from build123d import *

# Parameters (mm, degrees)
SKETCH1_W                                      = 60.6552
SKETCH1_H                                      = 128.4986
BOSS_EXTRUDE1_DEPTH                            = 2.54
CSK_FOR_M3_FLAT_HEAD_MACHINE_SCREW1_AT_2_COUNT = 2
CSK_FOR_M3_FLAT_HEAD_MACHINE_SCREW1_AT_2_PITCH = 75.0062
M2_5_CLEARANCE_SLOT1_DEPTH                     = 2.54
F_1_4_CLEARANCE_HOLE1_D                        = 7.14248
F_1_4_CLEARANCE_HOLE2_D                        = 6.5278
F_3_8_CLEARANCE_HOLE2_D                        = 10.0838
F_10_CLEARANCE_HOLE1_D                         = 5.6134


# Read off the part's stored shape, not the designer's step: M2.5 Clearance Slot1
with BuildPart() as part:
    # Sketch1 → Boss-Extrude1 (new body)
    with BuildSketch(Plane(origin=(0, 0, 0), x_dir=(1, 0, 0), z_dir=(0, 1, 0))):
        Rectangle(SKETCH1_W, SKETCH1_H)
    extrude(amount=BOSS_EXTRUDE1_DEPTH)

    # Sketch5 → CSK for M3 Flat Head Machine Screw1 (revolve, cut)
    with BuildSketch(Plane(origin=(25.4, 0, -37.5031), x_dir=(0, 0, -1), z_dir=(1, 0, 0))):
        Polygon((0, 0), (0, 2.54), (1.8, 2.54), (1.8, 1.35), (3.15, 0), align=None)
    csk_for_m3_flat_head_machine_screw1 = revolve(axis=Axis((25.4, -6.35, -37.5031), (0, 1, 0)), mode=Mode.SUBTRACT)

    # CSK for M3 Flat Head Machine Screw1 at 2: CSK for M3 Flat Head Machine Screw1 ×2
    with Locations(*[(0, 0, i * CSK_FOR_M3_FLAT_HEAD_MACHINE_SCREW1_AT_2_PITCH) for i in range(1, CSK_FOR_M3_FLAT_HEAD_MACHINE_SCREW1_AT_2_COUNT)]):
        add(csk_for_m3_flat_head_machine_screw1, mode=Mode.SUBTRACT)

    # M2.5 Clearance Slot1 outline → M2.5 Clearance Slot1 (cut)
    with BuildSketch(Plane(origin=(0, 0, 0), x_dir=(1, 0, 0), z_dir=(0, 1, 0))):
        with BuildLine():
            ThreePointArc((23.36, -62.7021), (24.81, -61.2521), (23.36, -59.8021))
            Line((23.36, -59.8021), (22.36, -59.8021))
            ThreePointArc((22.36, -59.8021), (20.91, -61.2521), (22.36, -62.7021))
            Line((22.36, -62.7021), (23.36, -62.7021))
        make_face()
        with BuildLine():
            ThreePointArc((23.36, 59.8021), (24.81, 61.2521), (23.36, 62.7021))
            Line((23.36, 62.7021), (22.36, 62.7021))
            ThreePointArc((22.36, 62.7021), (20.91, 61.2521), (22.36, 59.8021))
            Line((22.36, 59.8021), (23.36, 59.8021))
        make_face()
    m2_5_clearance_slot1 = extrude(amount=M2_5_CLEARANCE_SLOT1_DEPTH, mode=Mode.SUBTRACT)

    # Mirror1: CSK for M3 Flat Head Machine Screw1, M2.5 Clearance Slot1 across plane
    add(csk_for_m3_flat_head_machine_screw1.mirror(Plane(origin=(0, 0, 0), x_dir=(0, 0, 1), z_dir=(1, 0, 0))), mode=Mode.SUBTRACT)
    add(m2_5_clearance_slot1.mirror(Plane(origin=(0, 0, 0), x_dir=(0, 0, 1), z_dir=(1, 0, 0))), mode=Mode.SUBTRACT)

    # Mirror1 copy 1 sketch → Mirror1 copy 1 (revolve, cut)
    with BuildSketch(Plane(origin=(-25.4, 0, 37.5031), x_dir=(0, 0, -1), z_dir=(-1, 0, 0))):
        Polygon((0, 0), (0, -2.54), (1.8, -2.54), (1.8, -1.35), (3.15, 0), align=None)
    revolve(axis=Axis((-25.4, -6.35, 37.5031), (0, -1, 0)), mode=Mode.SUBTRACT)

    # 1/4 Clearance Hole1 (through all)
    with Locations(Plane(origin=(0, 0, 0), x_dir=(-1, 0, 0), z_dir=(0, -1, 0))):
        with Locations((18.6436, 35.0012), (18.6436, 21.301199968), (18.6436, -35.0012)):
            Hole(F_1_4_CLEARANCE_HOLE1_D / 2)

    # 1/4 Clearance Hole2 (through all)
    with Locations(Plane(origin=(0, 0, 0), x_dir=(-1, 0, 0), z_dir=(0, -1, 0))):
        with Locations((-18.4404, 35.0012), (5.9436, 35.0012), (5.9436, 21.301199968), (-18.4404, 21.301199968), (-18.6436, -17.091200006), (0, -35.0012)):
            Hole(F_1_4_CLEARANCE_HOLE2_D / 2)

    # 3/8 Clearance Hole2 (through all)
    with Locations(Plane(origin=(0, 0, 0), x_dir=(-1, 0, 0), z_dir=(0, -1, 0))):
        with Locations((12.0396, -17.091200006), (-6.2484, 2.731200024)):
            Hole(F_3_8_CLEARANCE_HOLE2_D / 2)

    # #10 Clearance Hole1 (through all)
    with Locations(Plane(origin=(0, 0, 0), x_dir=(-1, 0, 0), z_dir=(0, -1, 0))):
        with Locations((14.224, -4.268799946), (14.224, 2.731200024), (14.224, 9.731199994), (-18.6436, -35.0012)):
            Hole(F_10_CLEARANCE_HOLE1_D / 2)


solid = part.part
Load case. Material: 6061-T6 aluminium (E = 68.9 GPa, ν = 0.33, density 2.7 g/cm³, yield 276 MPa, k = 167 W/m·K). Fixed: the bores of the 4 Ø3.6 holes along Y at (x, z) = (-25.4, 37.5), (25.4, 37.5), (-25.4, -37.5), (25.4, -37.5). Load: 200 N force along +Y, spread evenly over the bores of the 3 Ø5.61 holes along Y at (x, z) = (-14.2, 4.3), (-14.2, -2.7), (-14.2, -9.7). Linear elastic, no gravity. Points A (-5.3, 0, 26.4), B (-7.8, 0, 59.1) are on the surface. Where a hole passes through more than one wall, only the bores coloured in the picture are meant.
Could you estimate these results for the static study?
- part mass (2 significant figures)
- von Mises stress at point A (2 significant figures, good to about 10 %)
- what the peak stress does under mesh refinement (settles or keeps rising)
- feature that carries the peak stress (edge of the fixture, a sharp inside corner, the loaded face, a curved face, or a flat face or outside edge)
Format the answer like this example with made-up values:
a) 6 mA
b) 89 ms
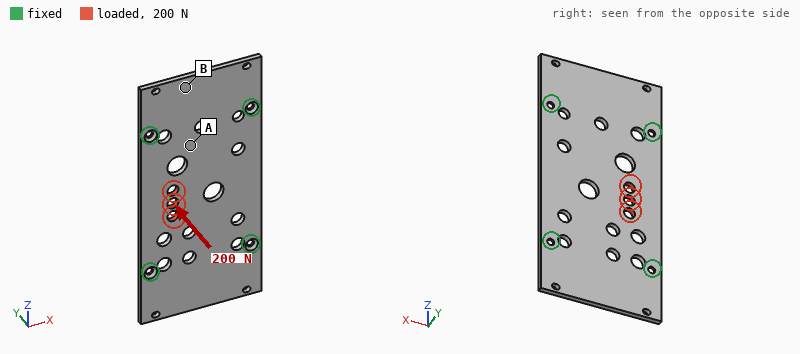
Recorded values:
a) 49 g
b) 19 MPa
c) keeps rising
d) edge of the fixture
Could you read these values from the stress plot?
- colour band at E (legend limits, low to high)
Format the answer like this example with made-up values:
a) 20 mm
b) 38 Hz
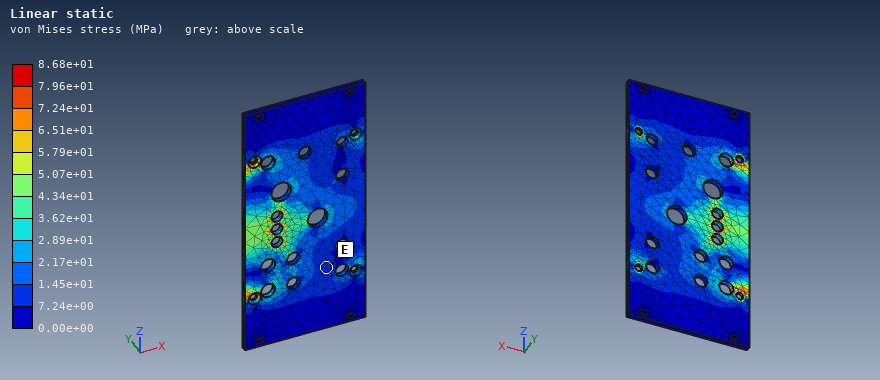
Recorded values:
a) 7.24e+00 to 1.45e+01 MPa
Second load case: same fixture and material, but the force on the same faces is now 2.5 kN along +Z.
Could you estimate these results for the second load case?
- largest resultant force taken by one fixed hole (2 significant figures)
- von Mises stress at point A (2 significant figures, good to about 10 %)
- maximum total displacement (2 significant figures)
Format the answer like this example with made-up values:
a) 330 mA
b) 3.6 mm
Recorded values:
a) 860 N
b) 8.1 MPa
c) 20 µm
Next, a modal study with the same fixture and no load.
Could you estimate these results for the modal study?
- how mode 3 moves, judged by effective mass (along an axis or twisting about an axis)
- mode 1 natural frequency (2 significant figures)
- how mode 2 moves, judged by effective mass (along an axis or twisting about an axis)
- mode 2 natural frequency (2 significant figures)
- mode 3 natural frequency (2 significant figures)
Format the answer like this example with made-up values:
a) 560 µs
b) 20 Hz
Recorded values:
a) along Y
b) 1600 Hz
c) twisting about X
d) 1900 Hz
e) 2000 Hz
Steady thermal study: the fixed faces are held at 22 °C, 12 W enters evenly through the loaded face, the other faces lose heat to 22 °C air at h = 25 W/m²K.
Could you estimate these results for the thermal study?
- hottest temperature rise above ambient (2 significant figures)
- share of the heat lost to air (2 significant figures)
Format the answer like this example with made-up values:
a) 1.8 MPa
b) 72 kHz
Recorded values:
a) 18 K
b) 16 %
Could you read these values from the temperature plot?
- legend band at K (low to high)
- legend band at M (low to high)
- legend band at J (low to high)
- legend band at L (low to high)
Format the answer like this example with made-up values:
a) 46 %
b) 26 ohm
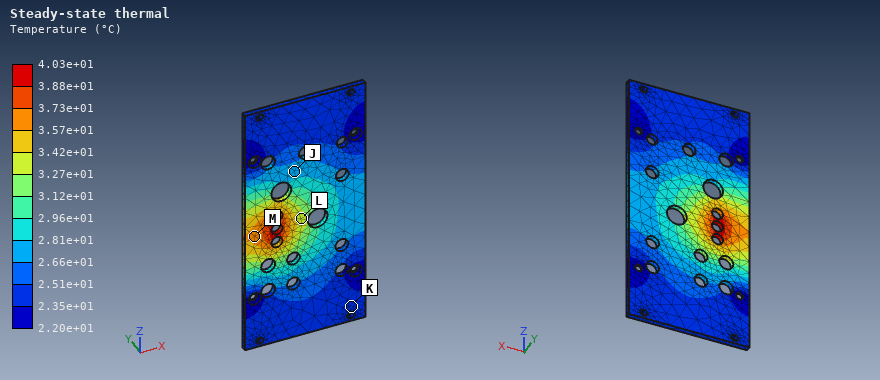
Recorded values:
a) 2.35e+01 to 2.51e+01 °C
b) 3.57e+01 to 3.73e+01 °C
c) 2.66e+01 to 2.81e+01 °C
d) 3.27e+01 to 3.42e+01 °C
